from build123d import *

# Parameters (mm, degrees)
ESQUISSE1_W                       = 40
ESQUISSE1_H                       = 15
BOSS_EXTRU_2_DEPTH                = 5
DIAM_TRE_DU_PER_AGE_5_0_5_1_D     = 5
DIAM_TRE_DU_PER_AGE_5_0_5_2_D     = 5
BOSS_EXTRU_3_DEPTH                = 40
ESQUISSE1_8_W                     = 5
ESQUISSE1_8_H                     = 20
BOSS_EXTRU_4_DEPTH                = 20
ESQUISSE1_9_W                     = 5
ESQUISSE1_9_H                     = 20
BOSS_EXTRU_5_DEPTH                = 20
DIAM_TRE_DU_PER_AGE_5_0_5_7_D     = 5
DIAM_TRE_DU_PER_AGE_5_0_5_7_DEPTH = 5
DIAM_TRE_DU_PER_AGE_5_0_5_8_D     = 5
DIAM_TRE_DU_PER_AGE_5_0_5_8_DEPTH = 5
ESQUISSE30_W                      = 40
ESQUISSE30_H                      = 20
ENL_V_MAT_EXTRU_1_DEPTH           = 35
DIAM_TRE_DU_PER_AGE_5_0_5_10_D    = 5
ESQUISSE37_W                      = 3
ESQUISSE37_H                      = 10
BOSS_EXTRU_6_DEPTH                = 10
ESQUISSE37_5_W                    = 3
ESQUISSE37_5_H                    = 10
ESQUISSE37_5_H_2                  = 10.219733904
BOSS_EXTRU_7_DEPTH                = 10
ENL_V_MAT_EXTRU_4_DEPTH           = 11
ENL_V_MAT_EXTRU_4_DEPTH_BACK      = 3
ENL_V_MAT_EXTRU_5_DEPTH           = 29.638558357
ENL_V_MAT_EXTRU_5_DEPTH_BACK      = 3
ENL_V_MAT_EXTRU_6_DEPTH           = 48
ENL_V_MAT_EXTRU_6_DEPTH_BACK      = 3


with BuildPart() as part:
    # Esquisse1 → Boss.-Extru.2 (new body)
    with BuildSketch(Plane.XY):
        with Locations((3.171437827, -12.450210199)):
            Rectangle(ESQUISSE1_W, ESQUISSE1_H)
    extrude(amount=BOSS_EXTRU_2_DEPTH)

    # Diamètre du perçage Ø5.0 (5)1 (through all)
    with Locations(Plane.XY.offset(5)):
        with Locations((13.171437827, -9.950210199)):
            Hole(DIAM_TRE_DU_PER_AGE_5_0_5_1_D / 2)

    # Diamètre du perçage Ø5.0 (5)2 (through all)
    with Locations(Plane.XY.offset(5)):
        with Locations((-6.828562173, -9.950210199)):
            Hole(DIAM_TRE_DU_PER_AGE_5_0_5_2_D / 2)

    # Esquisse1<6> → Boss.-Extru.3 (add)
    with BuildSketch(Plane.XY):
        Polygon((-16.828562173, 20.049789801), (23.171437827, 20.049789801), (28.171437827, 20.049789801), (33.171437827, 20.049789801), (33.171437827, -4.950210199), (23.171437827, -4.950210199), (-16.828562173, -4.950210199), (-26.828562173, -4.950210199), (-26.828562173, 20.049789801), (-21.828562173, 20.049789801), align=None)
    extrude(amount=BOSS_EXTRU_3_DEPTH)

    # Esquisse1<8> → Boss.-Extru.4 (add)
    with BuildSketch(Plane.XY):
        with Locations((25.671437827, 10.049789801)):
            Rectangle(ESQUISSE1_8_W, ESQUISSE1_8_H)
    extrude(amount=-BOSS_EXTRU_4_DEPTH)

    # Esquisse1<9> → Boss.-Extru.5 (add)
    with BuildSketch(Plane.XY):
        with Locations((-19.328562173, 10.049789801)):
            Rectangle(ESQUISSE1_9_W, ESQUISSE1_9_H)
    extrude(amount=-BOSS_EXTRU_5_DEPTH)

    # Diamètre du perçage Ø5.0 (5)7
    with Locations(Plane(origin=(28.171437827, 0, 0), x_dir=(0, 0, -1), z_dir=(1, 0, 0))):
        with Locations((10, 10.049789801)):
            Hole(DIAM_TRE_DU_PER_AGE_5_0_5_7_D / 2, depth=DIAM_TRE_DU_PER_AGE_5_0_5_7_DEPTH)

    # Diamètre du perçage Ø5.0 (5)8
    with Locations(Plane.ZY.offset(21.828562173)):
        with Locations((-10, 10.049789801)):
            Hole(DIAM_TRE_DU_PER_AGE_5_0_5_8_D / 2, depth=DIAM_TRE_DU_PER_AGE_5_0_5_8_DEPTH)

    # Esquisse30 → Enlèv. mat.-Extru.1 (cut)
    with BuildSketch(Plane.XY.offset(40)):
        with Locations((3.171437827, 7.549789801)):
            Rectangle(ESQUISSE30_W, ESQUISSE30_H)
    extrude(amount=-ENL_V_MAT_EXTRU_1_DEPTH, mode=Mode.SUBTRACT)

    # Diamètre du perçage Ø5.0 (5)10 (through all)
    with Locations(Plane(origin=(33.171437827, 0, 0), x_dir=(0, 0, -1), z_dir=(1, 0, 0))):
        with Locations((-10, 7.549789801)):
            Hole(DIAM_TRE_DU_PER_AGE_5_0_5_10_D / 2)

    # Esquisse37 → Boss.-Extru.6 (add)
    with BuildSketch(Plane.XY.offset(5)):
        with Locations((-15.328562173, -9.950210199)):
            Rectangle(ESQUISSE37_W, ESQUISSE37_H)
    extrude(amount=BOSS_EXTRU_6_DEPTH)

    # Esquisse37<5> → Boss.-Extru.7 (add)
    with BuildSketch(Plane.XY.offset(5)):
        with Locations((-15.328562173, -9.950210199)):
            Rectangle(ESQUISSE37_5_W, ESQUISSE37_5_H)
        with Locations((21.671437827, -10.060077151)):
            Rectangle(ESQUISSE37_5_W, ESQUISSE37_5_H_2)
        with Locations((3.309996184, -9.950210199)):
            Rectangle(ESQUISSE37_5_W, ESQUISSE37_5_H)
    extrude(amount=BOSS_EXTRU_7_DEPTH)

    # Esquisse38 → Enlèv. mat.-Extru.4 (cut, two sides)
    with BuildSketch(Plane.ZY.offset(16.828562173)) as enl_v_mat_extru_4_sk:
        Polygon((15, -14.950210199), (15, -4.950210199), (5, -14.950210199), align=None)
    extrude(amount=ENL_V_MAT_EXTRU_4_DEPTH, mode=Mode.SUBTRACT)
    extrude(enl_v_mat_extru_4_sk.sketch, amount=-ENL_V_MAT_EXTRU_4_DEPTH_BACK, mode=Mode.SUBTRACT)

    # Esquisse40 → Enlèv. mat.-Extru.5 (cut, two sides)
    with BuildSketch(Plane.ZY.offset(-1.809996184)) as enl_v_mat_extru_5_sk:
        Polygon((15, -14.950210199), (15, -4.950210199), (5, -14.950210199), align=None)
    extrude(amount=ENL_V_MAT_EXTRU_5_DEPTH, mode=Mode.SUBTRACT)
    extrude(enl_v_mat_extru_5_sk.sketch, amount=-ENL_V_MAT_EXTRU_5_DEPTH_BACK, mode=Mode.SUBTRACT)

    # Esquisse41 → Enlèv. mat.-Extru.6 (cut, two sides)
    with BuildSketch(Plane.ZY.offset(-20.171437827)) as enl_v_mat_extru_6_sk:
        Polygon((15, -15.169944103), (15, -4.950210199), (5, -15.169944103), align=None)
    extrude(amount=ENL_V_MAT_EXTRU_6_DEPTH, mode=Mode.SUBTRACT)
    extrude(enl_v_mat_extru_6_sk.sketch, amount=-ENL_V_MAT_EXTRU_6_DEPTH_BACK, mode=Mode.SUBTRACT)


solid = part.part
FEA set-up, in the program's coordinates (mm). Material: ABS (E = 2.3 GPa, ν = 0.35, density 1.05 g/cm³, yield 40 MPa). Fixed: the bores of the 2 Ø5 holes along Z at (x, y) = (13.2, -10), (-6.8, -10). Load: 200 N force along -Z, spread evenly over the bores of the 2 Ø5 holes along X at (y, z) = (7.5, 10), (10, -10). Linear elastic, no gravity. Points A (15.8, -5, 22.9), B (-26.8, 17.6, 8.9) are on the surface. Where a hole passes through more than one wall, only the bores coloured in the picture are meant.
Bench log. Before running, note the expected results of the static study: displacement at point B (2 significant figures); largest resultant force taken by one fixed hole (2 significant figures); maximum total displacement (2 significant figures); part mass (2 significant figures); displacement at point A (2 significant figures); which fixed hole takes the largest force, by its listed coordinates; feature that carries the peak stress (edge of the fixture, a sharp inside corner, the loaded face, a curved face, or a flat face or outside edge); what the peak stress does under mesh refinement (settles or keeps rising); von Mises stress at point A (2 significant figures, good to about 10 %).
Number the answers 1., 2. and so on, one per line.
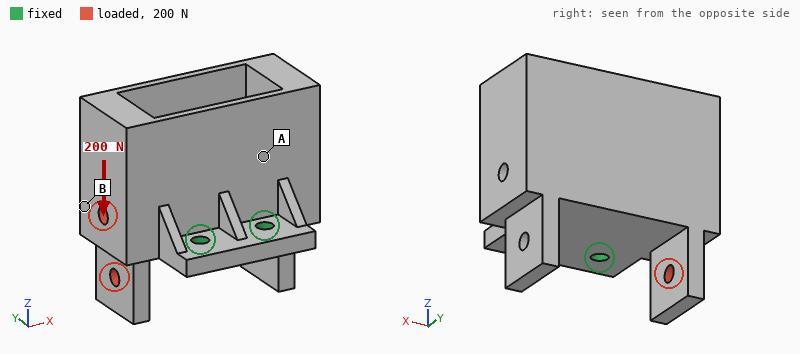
1. 0.67 mm
2. 290 N
3. 1.1 mm
4. 41 g
5. 0.24 mm
6. (-6.8, -10)
7. edge of the fixture
8. keeps rising
9. 3.5 MPa
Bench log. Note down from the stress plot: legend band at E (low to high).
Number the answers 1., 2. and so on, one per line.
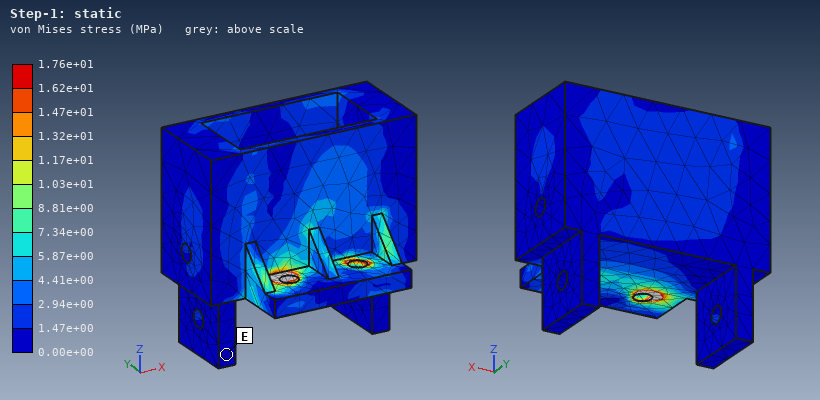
1. 0.00e+00 to 1.47e+00 MPa
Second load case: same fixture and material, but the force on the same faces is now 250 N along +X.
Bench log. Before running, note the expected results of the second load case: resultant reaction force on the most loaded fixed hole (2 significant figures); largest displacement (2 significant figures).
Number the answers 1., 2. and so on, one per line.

1. 230 N
2. 0.30 mm
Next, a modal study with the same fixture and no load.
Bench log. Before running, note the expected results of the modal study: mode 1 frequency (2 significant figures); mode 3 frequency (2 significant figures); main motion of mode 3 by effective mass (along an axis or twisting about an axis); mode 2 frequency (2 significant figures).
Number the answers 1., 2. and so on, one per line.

1. 440 Hz
2. 1400 Hz
3. along X
4. 720 Hz
